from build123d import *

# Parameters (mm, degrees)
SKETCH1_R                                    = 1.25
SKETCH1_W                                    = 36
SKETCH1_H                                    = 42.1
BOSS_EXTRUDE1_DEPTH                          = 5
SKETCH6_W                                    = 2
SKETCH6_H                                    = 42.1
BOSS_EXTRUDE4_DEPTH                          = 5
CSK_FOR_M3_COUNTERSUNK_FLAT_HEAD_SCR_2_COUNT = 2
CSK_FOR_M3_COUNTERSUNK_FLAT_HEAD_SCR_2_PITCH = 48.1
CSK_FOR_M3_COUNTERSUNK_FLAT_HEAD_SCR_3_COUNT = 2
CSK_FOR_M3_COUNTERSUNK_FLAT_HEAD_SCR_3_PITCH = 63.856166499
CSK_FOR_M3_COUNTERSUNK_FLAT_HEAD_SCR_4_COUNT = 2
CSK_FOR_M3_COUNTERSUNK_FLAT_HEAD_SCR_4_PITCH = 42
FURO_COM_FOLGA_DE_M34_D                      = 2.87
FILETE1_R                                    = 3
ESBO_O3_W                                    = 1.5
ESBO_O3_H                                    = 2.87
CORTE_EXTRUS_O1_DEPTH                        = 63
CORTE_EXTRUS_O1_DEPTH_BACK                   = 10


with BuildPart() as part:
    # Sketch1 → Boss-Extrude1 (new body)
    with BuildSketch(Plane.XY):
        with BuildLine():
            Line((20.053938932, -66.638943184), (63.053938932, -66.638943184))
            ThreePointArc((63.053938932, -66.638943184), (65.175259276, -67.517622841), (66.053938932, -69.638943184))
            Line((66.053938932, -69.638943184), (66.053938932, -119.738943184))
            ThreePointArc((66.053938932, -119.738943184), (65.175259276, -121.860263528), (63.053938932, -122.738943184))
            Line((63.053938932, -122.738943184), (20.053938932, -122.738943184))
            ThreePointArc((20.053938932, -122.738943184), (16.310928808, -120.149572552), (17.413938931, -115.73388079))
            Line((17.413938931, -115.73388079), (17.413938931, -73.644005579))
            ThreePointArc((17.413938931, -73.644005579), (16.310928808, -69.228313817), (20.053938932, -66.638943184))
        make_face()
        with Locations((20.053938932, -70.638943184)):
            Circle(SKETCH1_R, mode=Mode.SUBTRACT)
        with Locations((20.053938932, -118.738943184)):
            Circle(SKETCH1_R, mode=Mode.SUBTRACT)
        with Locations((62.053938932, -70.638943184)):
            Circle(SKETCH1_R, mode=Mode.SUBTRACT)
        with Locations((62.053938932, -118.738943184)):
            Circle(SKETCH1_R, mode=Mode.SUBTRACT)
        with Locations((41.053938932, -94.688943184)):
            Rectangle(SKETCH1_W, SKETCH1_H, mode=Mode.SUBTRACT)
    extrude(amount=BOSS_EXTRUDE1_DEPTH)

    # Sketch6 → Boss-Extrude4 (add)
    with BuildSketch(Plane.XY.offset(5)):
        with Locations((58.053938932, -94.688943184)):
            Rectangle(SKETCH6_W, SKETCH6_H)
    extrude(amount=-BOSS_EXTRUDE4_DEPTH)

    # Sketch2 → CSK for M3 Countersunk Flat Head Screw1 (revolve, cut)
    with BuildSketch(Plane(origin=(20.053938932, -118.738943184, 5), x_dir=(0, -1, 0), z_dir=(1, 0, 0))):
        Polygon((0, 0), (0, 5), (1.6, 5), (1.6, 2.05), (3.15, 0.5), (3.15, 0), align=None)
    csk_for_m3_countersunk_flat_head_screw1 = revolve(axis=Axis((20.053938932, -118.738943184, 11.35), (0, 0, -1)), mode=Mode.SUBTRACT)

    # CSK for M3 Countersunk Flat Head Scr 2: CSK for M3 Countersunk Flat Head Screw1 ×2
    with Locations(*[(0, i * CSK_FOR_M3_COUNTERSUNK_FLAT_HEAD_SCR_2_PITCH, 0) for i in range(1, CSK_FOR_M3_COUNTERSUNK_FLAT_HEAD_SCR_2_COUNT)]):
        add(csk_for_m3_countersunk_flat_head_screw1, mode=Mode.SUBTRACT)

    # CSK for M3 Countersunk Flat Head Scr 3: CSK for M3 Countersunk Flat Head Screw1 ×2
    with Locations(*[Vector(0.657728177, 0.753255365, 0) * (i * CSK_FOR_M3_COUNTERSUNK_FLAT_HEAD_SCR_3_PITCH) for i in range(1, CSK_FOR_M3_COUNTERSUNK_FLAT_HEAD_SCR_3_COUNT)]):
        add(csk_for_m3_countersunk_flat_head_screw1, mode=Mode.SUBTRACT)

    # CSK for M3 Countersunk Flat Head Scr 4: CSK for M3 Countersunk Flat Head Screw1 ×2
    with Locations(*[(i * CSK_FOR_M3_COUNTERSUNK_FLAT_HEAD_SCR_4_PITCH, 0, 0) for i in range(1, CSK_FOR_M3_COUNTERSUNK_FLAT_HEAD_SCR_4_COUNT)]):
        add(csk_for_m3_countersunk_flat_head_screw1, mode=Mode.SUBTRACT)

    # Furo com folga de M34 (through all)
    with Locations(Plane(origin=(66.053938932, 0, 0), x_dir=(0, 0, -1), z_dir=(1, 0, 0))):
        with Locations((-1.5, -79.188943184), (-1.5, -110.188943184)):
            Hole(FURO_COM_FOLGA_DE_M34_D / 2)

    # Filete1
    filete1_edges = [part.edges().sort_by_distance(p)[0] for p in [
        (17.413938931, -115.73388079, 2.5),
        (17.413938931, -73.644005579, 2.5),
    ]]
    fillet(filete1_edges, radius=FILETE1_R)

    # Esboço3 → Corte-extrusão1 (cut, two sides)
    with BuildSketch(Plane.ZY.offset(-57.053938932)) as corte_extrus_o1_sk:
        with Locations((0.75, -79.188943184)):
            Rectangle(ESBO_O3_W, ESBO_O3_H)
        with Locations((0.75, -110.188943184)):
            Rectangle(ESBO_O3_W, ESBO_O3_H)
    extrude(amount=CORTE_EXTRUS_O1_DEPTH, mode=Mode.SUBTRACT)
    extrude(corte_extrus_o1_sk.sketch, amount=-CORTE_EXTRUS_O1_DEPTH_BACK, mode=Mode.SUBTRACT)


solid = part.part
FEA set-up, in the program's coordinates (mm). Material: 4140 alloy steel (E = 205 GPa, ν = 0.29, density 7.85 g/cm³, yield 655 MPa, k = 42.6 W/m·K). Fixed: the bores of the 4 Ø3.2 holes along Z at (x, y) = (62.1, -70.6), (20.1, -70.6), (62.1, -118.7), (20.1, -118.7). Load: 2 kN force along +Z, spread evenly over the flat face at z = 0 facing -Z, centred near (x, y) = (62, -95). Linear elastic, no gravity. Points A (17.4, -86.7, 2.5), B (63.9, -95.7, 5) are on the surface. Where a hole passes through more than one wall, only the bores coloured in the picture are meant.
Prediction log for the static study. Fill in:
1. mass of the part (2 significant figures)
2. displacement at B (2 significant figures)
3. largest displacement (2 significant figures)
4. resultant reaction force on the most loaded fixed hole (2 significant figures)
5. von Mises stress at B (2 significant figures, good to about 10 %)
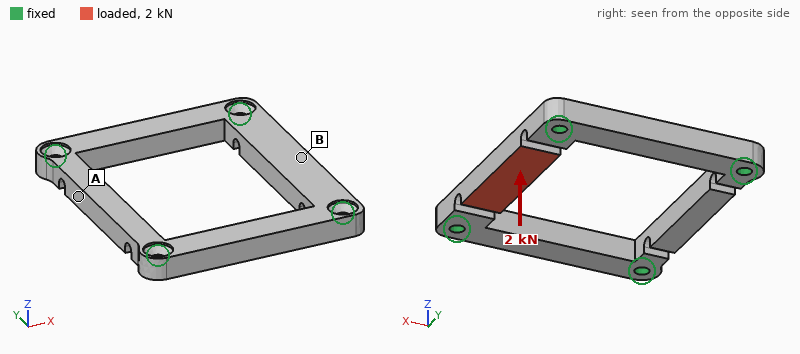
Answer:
47 g
68 µm
71 µm
1.0 kN
210 MPa
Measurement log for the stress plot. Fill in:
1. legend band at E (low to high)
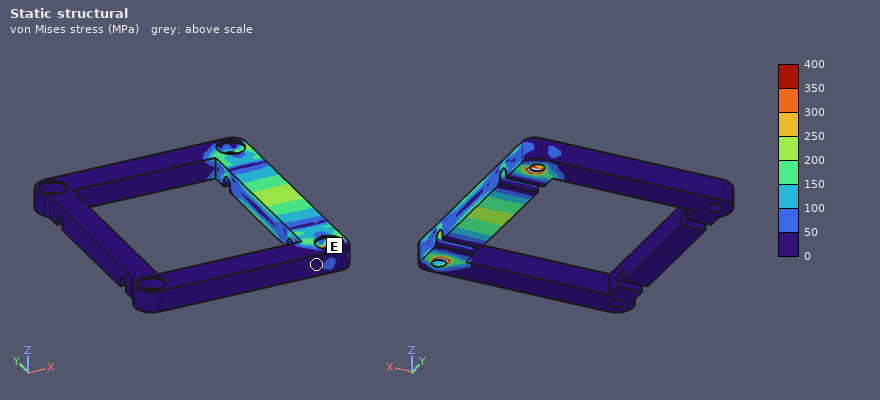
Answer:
0 to 50 MPa
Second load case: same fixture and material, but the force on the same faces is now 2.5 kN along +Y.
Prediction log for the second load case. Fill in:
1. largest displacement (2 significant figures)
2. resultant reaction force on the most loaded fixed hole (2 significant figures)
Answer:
13 µm
1.3 kN
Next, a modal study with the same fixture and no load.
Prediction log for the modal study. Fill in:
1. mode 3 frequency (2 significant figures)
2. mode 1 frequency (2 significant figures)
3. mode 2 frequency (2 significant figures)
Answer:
11 kHz
9200 Hz
9500 Hz
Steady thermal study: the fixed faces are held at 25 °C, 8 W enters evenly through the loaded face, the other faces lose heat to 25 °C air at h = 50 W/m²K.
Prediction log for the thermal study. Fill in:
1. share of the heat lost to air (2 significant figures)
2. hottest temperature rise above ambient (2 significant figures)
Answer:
18 %
43 K
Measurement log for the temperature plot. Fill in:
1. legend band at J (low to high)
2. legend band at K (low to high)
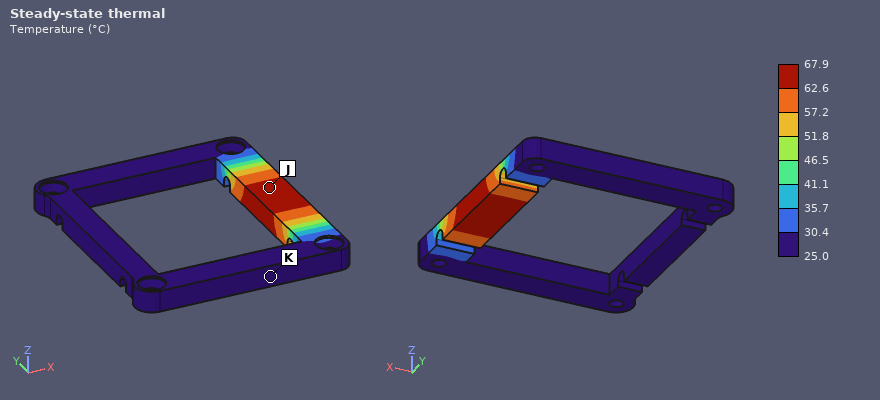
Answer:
62.6 to 67.9 °C
25.0 to 30.4 °C
